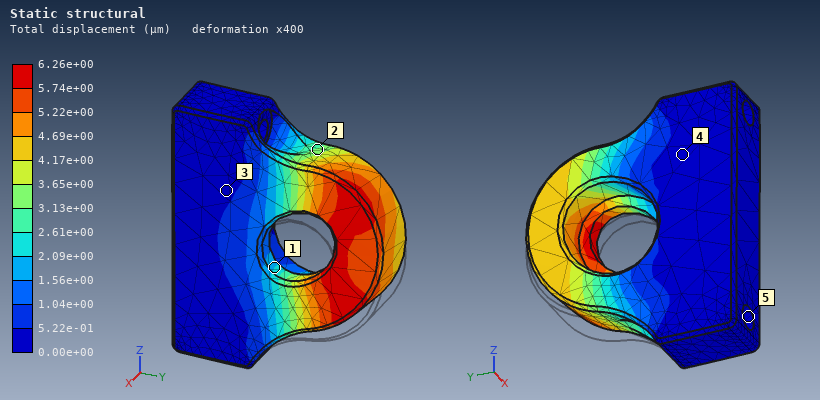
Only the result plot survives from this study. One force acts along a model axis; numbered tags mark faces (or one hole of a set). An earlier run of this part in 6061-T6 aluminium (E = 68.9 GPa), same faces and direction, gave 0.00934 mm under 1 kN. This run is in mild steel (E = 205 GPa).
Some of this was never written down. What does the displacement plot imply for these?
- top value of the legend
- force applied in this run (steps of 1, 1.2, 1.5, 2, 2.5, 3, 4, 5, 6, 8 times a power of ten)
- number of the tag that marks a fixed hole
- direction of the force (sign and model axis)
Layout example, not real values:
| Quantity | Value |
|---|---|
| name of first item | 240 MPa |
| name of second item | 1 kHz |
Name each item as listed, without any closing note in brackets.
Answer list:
| Quantity | Value |
|---|---|
| top value of the legend | 6.26e+00 µm |
| force applied in this run | 2 kN |
| number of the tag that marks a fixed hole | 5 |
| direction of the force | +Z |
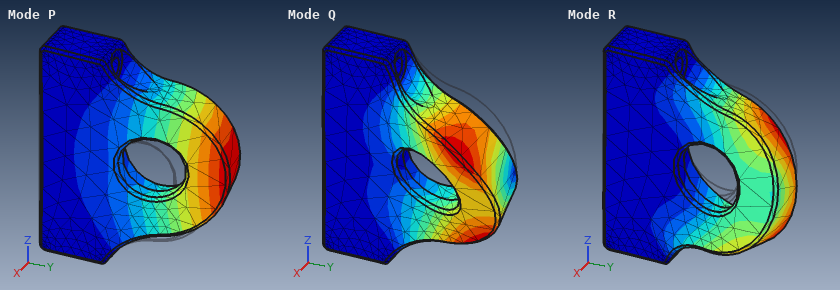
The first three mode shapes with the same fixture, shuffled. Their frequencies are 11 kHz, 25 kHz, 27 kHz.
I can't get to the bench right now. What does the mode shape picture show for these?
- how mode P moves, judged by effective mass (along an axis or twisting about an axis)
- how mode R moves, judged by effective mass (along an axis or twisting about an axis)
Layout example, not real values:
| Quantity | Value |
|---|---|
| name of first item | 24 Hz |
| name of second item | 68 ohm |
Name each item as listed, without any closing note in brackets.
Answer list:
| Quantity | Value |
|---|---|
| how mode P moves, judged by effective mass | along X |
| how mode R moves, judged by effective mass | along Z |
